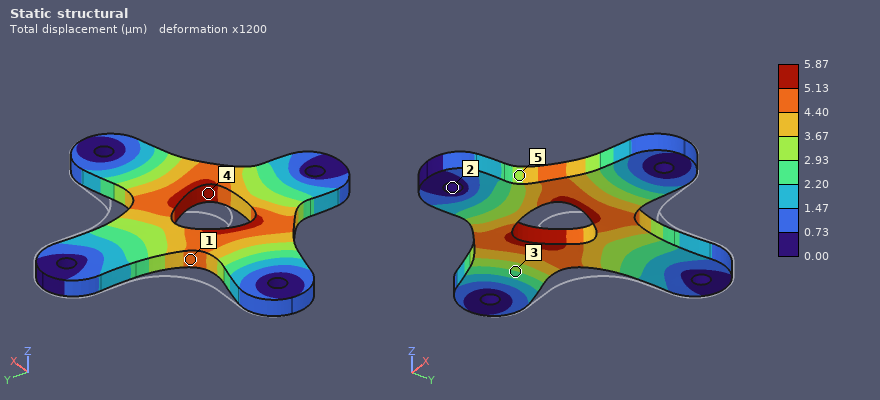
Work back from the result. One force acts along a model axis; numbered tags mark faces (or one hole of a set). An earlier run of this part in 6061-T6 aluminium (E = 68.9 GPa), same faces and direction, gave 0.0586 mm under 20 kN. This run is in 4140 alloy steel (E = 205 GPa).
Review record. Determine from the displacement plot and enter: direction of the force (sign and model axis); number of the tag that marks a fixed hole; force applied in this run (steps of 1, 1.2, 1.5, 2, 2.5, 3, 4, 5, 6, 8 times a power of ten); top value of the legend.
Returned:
-Y
2
6 kN
5.87 µm
